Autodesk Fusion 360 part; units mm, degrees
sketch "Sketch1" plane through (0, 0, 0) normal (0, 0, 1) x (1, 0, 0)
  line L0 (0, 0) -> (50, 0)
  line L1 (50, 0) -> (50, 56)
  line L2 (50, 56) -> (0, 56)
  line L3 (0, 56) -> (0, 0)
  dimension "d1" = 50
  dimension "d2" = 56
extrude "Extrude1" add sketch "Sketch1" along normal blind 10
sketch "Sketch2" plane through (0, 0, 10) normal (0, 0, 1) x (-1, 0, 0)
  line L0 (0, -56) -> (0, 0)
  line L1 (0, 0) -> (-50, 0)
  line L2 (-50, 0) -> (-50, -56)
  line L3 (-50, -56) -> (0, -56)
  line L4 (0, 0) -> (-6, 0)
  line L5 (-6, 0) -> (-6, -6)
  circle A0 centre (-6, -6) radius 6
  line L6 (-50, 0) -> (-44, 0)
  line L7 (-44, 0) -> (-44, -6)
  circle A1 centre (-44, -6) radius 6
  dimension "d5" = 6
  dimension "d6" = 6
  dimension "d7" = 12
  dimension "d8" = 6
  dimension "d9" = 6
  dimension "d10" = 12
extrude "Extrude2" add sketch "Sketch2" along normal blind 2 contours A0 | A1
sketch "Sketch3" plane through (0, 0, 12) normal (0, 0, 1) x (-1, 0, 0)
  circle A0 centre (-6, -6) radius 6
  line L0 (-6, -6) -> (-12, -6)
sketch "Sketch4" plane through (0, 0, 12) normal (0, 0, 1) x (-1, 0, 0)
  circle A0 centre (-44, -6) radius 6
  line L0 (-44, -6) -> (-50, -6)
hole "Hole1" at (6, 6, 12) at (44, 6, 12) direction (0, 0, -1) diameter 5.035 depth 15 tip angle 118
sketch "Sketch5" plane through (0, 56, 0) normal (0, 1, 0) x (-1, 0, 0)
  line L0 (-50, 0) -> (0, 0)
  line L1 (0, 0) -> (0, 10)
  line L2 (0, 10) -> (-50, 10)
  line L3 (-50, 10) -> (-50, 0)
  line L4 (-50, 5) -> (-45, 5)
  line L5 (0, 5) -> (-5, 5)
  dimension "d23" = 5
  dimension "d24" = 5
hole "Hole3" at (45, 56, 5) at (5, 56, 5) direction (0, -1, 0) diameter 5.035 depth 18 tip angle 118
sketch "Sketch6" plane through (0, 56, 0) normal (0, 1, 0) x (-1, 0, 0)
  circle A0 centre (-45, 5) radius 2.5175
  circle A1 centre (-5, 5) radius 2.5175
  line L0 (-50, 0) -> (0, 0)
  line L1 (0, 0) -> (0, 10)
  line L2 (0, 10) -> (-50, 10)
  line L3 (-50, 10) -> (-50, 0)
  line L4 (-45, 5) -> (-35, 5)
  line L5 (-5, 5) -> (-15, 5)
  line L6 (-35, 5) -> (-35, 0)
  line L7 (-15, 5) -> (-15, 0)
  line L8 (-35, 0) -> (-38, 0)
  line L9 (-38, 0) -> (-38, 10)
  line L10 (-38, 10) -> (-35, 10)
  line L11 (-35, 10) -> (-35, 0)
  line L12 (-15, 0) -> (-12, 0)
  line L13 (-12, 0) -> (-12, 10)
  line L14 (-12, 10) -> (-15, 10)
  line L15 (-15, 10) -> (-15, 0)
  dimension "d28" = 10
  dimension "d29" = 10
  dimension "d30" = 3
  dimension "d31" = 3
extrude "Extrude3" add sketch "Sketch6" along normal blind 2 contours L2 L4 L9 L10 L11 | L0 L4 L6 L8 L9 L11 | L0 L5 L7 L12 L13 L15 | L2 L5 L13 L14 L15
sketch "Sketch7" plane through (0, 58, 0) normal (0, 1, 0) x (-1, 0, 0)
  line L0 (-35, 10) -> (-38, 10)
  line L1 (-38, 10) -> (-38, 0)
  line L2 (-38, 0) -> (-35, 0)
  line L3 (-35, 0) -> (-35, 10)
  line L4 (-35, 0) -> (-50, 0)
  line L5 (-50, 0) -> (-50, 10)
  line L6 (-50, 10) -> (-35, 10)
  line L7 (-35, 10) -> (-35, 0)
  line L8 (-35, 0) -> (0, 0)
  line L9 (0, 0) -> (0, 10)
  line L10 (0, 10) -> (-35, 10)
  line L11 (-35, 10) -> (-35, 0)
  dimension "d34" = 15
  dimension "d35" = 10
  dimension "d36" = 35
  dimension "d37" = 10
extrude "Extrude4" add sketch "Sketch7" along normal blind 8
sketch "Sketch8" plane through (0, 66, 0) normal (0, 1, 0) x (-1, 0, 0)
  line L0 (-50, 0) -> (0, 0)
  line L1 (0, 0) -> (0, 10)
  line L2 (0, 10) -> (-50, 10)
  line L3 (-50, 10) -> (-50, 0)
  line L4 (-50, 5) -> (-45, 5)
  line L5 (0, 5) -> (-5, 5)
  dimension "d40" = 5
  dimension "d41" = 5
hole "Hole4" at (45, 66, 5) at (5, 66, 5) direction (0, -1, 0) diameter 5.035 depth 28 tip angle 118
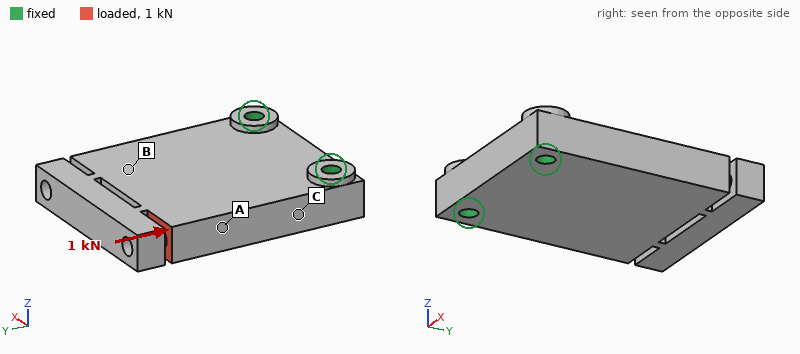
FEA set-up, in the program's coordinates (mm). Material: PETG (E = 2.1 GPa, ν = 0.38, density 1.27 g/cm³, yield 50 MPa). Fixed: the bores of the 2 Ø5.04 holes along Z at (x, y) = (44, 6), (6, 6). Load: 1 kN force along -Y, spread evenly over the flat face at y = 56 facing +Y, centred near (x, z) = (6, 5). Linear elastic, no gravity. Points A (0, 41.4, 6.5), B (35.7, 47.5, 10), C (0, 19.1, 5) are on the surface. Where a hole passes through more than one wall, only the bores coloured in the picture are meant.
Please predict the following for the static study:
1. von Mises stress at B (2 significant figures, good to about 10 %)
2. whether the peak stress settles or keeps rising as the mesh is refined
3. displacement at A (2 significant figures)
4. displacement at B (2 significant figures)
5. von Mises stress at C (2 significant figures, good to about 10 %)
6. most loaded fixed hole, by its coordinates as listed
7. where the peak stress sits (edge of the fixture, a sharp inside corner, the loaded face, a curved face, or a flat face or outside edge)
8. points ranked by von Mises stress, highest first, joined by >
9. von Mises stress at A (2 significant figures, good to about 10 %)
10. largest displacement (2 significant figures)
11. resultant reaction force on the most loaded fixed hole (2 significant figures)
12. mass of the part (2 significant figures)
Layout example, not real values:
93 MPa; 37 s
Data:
0.99 MPa; keeps rising; 0.15 mm; 0.074 mm; 7.3 MPa; (6, 6); edge of the fixture; A > C > B; 10 MPa; 0.25 mm; 990 N; 39 g
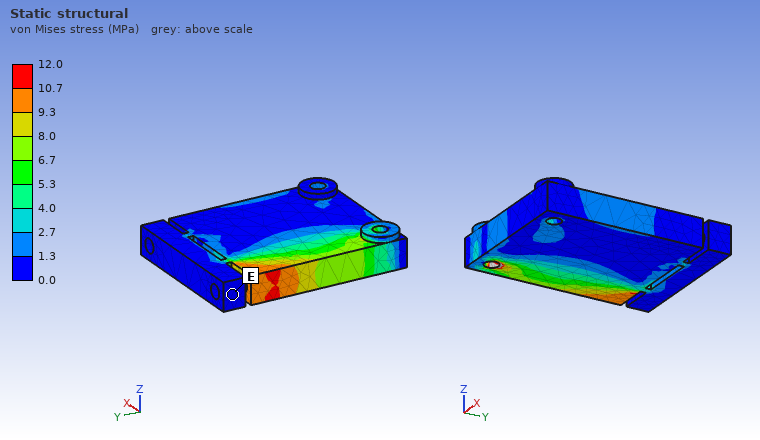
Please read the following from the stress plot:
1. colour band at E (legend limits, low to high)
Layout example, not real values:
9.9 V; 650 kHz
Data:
0.0 to 1.3 MPa
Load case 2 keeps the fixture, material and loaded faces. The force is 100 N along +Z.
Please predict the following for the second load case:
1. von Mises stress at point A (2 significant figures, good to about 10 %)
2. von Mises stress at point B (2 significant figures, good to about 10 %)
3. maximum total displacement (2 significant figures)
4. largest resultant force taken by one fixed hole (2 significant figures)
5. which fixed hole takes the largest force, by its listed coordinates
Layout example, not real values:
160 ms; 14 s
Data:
3.3 MPa; 1.6 MPa; 0.87 mm; 98 N; (6, 6)
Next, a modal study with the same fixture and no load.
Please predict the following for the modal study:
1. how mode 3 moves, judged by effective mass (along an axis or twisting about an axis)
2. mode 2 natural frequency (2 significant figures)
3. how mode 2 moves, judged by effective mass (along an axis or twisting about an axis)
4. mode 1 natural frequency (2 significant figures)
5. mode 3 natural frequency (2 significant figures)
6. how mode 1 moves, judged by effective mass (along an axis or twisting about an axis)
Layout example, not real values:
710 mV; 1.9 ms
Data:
along X; 1500 Hz; twisting about Y; 570 Hz; 2100 Hz; along Z
